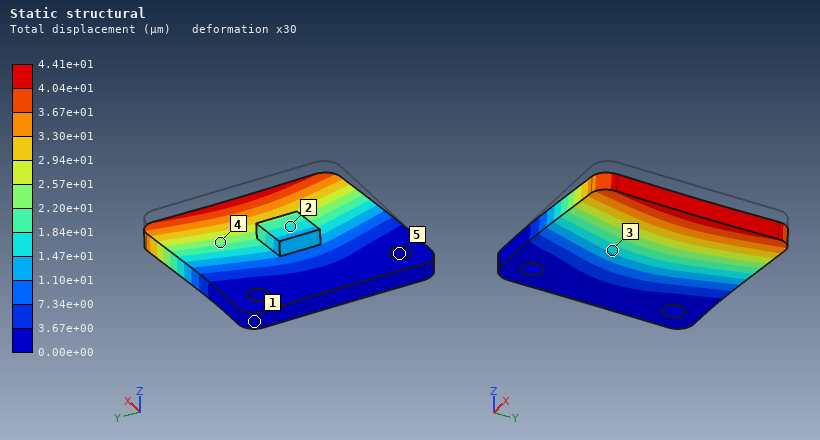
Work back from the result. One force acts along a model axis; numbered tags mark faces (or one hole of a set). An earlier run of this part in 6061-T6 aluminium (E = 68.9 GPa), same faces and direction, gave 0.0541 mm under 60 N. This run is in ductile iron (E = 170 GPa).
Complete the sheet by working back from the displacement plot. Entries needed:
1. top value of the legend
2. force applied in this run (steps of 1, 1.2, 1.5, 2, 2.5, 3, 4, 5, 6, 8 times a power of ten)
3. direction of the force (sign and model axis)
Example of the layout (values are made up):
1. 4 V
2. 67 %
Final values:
1. 4.41e+01 µm
2. 120 N
3. -Z
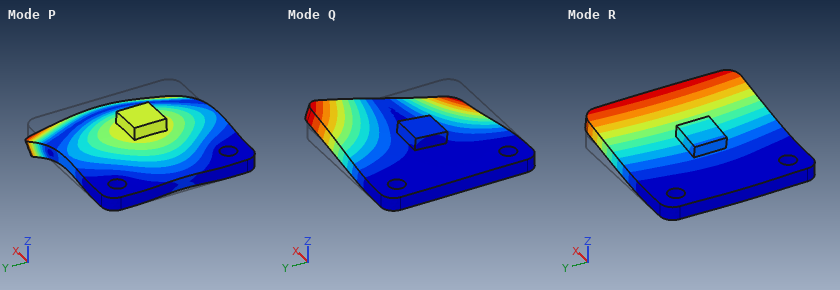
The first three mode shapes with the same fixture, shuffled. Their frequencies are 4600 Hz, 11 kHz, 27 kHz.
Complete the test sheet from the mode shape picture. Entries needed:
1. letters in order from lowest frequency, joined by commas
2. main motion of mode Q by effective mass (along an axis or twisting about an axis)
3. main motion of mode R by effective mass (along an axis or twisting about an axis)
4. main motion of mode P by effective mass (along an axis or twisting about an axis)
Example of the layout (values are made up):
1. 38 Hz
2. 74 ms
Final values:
1. R, Q, P
2. twisting about X
3. along Z
4. along Z
